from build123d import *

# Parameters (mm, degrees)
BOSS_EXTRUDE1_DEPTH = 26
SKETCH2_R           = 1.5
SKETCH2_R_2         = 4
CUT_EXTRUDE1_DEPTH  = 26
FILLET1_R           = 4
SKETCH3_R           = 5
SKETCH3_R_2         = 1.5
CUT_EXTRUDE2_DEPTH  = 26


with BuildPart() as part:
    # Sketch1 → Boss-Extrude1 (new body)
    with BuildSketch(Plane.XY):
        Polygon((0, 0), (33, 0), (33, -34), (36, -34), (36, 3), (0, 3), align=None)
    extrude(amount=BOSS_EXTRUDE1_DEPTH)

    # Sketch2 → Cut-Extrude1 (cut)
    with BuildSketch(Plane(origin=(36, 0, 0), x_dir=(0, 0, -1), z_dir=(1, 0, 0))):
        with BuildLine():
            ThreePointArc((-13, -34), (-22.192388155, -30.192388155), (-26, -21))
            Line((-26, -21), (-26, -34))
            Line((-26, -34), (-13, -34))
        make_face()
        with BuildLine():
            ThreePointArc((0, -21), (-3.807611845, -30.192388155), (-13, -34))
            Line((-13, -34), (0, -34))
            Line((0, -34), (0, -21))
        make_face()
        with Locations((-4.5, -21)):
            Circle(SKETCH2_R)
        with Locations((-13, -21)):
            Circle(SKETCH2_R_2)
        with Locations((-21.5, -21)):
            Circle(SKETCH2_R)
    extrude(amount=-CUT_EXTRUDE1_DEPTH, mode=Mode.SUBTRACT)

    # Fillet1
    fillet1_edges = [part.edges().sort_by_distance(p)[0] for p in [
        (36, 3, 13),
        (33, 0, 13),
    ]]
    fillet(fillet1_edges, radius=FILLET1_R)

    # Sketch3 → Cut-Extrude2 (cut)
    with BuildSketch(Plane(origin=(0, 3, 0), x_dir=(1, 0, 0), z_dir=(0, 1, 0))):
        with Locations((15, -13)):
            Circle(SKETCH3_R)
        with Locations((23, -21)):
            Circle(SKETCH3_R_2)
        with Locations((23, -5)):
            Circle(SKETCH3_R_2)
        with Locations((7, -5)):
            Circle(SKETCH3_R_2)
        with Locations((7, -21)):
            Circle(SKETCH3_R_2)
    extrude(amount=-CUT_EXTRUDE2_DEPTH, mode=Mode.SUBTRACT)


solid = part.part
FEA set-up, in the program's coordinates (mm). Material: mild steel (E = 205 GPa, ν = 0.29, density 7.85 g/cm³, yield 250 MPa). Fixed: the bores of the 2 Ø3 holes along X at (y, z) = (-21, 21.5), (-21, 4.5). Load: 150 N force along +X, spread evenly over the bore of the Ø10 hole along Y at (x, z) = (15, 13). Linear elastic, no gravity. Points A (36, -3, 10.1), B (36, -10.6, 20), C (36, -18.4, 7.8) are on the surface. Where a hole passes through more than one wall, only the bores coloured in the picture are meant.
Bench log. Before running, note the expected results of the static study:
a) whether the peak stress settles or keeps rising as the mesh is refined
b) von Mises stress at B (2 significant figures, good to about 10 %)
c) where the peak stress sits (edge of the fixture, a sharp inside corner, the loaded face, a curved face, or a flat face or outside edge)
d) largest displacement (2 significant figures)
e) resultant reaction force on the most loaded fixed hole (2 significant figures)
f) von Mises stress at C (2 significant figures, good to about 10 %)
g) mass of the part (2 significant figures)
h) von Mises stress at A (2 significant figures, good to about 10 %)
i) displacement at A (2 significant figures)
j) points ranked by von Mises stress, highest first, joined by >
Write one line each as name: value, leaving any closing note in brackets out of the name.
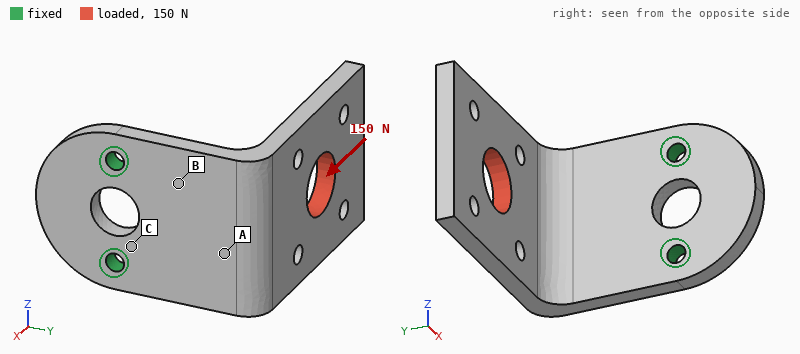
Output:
whether the peak stress settles or keeps rising as the mesh is refined: keeps rising
von Mises stress at B: 44 MPa
where the peak stress sits: edge of the fixture
largest displacement: 0.13 mm
resultant reaction force on the most loaded fixed hole: 75 N
von Mises stress at C: 87 MPa
mass of the part: 37 g
von Mises stress at A: 16 MPa
displacement at A: 0.038 mm
points ranked by von Mises stress, highest first, joined by >: C > B > A
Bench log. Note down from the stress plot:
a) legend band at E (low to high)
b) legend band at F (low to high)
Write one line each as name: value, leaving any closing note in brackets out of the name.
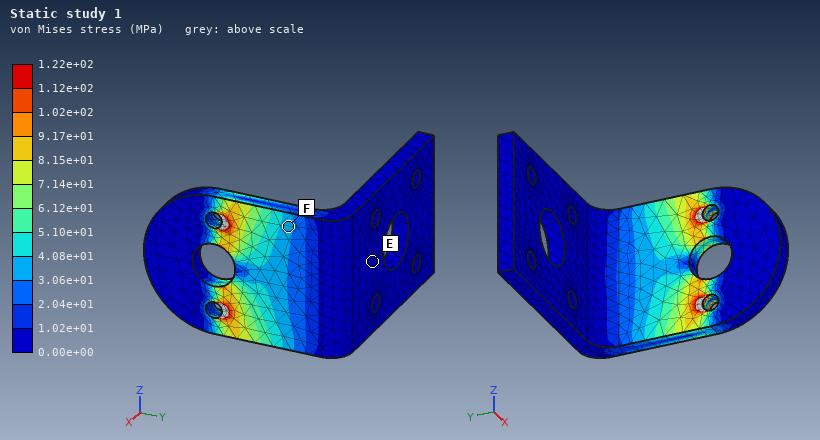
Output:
legend band at E: 0.00e+00 to 1.02e+01 MPa
legend band at F: 3.06e+01 to 4.08e+01 MPa
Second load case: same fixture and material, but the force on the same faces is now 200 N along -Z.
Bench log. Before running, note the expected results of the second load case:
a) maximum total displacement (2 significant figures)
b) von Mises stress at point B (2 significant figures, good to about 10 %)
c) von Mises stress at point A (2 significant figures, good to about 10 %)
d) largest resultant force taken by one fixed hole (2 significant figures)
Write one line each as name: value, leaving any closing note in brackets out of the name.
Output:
maximum total displacement: 100 µm
von Mises stress at point B: 58 MPa
von Mises stress at point A: 46 MPa
largest resultant force taken by one fixed hole: 320 N
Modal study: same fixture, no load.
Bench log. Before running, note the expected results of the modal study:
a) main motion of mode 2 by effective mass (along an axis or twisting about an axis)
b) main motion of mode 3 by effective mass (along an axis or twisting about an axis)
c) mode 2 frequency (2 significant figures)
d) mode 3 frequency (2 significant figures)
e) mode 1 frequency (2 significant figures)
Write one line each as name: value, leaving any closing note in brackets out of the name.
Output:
main motion of mode 2 by effective mass: along Z
main motion of mode 3 by effective mass: along X
mode 2 frequency: 2000 Hz
mode 3 frequency: 3200 Hz
mode 1 frequency: 1100 Hz
